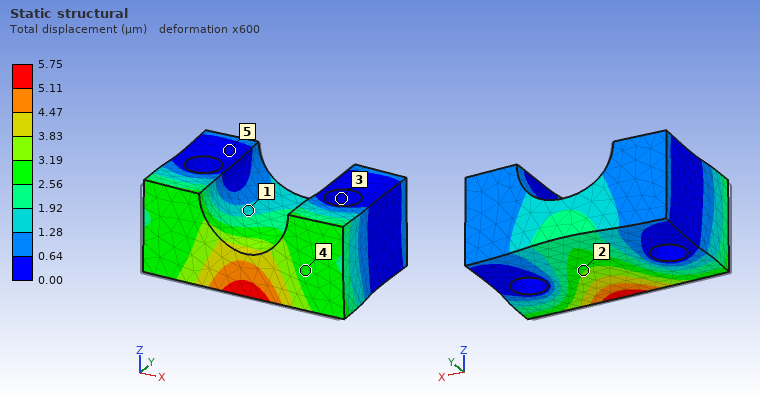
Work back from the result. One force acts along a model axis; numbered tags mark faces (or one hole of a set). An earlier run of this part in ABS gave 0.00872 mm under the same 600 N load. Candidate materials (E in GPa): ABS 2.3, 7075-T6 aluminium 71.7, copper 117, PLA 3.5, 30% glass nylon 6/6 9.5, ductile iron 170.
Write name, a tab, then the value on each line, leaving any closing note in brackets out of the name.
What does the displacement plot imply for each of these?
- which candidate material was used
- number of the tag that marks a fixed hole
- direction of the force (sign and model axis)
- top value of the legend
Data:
which candidate material was used	PLA
number of the tag that marks a fixed hole	3
direction of the force	+Y
top value of the legend	5.75 µm
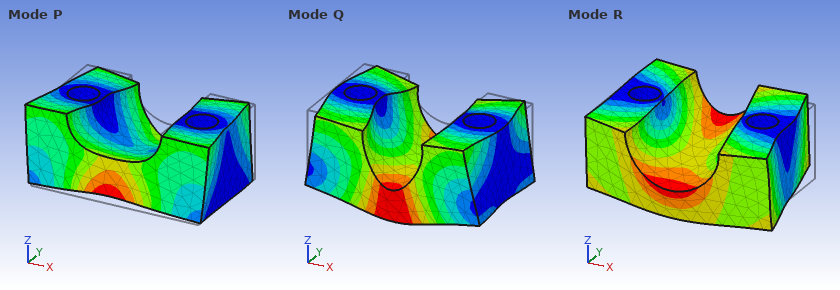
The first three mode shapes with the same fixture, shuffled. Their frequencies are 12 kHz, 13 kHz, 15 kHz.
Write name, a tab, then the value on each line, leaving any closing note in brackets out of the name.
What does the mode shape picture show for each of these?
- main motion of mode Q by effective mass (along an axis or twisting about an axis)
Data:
main motion of mode Q by effective mass	along Z
